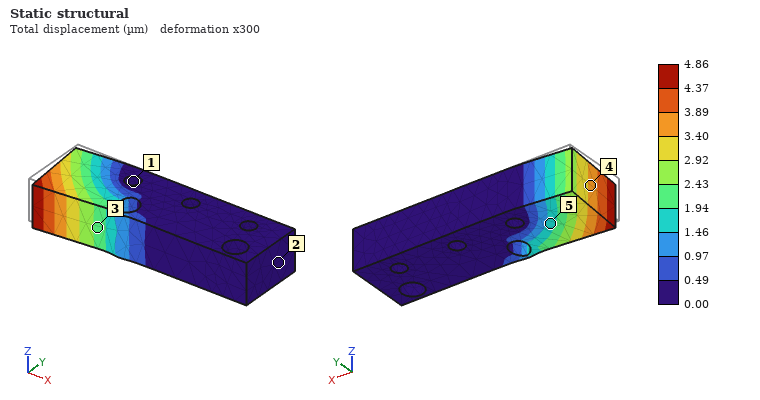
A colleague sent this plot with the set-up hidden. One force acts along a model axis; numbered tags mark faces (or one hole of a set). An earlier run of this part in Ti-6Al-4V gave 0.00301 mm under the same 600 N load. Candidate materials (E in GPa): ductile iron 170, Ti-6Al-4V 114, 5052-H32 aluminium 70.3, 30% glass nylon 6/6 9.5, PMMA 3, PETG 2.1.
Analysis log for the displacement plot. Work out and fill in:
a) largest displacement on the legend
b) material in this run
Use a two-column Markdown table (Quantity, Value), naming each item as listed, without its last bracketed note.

| Quantity | Value |
|---|---|
| largest displacement on the legend | 4.86 µm |
| material in this run | 5052-H32 aluminium |
